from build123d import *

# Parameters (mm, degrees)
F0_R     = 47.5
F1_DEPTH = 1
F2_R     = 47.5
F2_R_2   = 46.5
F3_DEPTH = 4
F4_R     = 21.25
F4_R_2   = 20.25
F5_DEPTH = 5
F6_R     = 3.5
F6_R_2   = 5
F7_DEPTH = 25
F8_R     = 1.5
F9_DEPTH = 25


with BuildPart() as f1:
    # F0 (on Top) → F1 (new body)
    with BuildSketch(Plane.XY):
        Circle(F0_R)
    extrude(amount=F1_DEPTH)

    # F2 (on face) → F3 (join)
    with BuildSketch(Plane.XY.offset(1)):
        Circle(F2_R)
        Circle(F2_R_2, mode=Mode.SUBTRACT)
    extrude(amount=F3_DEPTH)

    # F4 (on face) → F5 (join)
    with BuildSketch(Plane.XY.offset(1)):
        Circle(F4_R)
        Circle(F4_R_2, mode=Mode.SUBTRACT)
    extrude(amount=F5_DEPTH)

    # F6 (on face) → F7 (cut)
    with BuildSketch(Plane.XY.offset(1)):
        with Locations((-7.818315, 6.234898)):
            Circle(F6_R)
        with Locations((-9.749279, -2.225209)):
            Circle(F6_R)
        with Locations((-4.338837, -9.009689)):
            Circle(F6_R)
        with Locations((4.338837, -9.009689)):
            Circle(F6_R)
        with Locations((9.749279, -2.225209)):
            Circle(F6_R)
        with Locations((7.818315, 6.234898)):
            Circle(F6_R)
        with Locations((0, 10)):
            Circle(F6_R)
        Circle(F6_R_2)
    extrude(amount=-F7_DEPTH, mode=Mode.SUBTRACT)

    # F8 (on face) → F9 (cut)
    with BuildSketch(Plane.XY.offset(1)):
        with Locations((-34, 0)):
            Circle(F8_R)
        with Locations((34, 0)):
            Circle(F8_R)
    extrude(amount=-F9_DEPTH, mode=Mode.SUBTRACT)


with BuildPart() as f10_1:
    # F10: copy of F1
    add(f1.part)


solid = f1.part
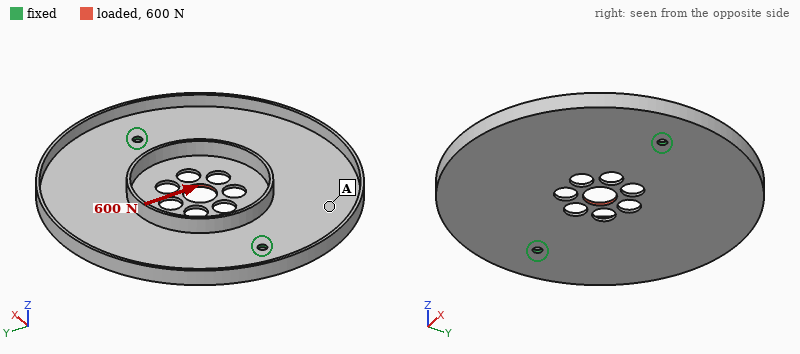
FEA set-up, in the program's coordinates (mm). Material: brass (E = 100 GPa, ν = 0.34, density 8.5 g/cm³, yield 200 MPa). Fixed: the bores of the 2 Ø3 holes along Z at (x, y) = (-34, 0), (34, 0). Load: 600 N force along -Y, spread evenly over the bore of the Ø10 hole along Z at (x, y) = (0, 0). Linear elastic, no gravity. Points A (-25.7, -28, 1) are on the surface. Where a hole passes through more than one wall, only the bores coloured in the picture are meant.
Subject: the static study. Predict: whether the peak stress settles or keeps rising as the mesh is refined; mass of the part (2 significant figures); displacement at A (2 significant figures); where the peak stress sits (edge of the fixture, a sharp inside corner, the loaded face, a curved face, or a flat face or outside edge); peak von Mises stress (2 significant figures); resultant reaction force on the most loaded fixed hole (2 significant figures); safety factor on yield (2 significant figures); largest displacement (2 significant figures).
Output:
settles
73 g
3.1 µm
a curved face
100 MPa
300 N
1.9
12 µm
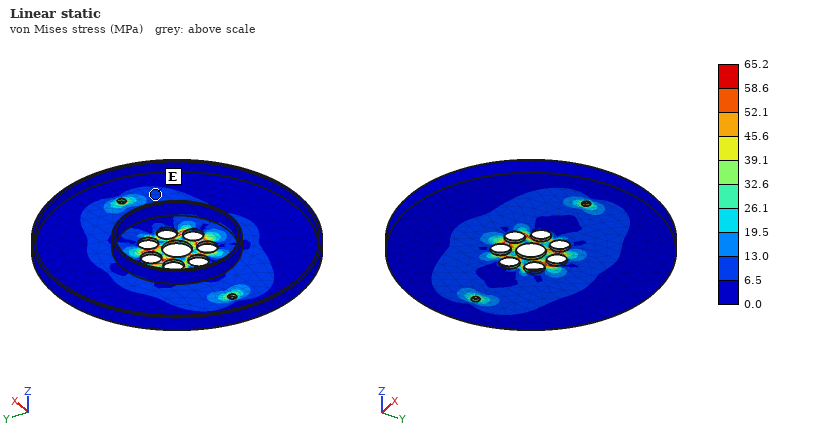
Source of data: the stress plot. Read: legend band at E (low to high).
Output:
6.5 to 13.0 MPa
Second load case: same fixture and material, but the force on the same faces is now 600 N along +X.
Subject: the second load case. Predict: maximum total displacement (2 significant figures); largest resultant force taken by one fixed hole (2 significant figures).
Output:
10 µm
300 N
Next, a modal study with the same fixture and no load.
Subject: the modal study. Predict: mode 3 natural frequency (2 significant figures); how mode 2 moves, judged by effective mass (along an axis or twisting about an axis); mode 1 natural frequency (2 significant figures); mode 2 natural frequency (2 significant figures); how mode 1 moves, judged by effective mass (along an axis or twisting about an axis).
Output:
820 Hz
along Z
260 Hz
530 Hz
twisting about X
